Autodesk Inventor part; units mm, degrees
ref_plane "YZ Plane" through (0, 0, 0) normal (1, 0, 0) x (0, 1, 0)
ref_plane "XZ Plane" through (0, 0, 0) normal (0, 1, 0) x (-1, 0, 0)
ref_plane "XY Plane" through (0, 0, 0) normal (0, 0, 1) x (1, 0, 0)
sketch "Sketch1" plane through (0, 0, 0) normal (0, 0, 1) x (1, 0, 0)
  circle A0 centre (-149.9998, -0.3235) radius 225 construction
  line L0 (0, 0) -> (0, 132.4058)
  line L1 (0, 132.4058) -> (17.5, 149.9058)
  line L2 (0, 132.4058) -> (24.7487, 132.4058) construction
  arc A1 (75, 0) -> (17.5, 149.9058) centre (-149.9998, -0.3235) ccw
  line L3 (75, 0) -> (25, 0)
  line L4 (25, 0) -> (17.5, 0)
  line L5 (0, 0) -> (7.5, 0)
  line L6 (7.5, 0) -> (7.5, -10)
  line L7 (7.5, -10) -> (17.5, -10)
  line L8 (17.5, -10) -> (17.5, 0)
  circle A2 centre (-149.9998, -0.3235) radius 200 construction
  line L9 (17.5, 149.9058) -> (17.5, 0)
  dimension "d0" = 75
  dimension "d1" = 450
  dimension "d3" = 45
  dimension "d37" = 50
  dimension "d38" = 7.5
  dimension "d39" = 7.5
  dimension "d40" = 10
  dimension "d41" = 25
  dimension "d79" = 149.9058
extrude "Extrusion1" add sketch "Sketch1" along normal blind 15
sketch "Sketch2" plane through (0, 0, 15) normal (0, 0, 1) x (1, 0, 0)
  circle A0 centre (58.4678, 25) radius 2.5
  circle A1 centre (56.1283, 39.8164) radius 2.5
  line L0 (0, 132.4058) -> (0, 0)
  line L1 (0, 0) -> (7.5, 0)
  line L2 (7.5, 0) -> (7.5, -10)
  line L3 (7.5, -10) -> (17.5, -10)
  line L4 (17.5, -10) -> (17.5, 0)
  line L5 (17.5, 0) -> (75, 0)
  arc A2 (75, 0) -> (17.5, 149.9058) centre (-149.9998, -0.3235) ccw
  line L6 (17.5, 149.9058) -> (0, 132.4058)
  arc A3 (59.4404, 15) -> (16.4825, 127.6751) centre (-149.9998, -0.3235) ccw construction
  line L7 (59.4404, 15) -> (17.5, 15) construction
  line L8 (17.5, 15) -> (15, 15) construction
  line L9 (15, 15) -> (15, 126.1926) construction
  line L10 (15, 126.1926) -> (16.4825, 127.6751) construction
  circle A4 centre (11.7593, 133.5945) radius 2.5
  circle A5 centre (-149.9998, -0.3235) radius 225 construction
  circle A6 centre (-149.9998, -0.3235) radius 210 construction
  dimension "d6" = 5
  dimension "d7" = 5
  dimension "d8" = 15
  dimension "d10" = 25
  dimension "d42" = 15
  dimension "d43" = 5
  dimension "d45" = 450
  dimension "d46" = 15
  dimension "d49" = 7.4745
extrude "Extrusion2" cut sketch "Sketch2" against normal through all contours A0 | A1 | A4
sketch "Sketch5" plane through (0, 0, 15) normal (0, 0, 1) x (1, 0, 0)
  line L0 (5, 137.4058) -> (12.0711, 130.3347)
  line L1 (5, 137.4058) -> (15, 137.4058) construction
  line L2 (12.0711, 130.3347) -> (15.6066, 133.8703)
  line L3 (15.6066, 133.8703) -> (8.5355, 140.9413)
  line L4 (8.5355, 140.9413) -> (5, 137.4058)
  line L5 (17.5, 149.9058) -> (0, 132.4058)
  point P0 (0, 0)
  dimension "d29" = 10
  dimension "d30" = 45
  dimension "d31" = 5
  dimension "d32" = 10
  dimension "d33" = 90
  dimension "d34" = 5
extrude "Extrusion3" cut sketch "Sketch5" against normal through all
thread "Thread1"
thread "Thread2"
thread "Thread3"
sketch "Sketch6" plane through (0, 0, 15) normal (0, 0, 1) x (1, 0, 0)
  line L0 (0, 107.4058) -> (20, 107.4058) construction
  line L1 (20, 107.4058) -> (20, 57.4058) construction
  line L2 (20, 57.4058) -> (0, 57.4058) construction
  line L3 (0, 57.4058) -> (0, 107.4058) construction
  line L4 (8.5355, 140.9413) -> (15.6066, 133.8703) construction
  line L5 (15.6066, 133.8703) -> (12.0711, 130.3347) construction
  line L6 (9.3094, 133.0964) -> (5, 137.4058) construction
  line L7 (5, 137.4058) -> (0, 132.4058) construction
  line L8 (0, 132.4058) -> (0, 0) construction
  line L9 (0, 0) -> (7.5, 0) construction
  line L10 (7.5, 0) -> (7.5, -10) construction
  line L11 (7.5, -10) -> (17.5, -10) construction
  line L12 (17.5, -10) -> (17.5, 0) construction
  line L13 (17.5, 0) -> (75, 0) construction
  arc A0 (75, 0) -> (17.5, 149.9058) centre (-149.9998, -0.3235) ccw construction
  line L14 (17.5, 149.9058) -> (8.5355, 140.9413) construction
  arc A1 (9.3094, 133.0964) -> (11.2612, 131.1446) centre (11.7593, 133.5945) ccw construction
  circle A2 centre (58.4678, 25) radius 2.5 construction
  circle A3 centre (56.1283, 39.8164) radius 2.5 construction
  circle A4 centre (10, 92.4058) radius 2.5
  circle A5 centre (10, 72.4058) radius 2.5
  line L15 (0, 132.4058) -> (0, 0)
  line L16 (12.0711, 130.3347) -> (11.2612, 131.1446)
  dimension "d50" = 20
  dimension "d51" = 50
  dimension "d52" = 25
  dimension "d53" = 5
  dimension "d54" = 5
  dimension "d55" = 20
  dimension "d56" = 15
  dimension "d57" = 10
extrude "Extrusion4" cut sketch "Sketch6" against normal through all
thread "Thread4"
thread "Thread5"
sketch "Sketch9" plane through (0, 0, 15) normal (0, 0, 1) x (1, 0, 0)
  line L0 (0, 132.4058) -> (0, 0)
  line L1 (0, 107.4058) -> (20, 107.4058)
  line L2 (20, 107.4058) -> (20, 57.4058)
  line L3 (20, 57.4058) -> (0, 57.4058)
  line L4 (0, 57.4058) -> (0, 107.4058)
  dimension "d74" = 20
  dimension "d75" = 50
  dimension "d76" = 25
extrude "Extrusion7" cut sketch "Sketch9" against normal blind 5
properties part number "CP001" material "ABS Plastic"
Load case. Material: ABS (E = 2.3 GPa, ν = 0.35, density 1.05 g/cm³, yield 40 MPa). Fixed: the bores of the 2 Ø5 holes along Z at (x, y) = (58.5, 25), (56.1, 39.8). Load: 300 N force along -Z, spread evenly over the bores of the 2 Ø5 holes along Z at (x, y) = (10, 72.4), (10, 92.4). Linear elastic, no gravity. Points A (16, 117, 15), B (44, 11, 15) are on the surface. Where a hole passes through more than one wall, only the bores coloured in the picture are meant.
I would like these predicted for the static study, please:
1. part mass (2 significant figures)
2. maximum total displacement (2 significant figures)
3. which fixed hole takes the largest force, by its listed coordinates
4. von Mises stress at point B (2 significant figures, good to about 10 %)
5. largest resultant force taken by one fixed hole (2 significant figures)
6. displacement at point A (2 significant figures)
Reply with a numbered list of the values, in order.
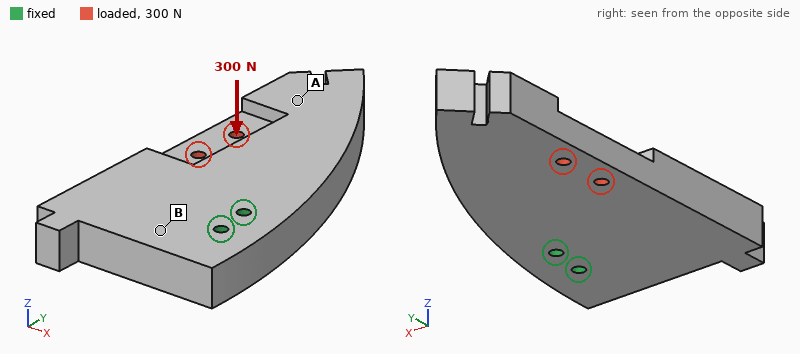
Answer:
1. 130 g
2. 1.6 mm
3. (56.1, 39.8)
4. 2.9 MPa
5. 600 N
6. 1.2 mm
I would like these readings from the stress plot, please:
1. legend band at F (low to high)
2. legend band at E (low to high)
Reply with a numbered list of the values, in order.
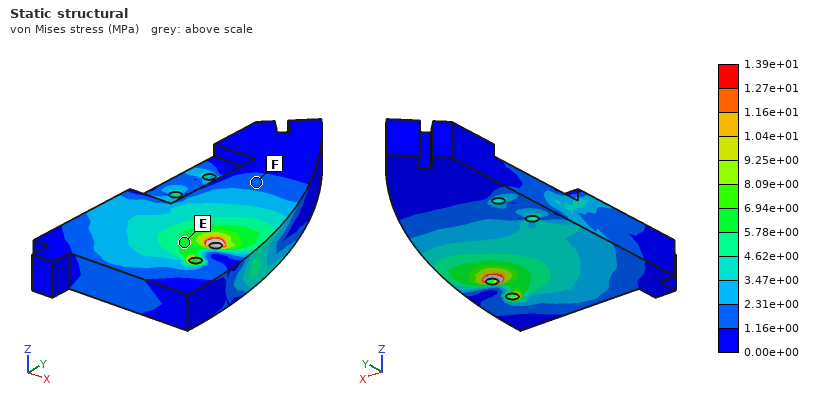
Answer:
1. 1.16e+00 to 2.31e+00 MPa
2. 5.78e+00 to 6.94e+00 MPa
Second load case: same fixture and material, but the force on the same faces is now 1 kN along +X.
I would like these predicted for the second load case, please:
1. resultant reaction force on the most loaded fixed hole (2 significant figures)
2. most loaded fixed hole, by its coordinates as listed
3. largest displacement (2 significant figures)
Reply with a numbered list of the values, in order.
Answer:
1. 3.1 kN
2. (56.1, 39.8)
3. 1.1 mm
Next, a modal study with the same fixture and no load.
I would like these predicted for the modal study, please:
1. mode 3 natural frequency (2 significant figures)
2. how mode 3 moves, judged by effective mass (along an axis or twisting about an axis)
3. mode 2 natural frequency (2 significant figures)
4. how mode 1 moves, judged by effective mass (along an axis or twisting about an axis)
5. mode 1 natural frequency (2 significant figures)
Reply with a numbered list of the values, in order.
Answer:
1. 840 Hz
2. along Z
3. 600 Hz
4. along Z
5. 320 Hz
